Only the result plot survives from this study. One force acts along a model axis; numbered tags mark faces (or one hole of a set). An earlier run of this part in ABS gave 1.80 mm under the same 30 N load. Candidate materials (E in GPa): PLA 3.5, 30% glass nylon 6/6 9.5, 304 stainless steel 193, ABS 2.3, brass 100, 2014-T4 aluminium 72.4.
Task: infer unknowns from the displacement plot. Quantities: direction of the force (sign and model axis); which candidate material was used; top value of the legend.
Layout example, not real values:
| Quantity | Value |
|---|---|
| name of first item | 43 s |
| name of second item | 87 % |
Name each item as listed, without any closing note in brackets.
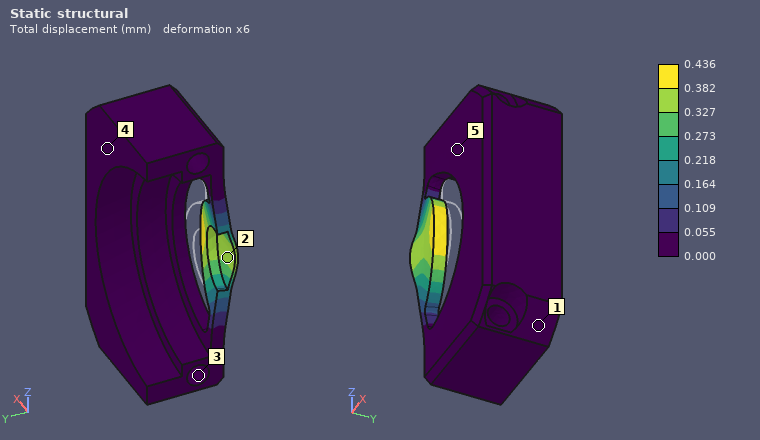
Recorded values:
| Quantity | Value |
|---|---|
| direction of the force | -Y |
| which candidate material was used | 30% glass nylon 6/6 |
| top value of the legend | 0.436 mm |
